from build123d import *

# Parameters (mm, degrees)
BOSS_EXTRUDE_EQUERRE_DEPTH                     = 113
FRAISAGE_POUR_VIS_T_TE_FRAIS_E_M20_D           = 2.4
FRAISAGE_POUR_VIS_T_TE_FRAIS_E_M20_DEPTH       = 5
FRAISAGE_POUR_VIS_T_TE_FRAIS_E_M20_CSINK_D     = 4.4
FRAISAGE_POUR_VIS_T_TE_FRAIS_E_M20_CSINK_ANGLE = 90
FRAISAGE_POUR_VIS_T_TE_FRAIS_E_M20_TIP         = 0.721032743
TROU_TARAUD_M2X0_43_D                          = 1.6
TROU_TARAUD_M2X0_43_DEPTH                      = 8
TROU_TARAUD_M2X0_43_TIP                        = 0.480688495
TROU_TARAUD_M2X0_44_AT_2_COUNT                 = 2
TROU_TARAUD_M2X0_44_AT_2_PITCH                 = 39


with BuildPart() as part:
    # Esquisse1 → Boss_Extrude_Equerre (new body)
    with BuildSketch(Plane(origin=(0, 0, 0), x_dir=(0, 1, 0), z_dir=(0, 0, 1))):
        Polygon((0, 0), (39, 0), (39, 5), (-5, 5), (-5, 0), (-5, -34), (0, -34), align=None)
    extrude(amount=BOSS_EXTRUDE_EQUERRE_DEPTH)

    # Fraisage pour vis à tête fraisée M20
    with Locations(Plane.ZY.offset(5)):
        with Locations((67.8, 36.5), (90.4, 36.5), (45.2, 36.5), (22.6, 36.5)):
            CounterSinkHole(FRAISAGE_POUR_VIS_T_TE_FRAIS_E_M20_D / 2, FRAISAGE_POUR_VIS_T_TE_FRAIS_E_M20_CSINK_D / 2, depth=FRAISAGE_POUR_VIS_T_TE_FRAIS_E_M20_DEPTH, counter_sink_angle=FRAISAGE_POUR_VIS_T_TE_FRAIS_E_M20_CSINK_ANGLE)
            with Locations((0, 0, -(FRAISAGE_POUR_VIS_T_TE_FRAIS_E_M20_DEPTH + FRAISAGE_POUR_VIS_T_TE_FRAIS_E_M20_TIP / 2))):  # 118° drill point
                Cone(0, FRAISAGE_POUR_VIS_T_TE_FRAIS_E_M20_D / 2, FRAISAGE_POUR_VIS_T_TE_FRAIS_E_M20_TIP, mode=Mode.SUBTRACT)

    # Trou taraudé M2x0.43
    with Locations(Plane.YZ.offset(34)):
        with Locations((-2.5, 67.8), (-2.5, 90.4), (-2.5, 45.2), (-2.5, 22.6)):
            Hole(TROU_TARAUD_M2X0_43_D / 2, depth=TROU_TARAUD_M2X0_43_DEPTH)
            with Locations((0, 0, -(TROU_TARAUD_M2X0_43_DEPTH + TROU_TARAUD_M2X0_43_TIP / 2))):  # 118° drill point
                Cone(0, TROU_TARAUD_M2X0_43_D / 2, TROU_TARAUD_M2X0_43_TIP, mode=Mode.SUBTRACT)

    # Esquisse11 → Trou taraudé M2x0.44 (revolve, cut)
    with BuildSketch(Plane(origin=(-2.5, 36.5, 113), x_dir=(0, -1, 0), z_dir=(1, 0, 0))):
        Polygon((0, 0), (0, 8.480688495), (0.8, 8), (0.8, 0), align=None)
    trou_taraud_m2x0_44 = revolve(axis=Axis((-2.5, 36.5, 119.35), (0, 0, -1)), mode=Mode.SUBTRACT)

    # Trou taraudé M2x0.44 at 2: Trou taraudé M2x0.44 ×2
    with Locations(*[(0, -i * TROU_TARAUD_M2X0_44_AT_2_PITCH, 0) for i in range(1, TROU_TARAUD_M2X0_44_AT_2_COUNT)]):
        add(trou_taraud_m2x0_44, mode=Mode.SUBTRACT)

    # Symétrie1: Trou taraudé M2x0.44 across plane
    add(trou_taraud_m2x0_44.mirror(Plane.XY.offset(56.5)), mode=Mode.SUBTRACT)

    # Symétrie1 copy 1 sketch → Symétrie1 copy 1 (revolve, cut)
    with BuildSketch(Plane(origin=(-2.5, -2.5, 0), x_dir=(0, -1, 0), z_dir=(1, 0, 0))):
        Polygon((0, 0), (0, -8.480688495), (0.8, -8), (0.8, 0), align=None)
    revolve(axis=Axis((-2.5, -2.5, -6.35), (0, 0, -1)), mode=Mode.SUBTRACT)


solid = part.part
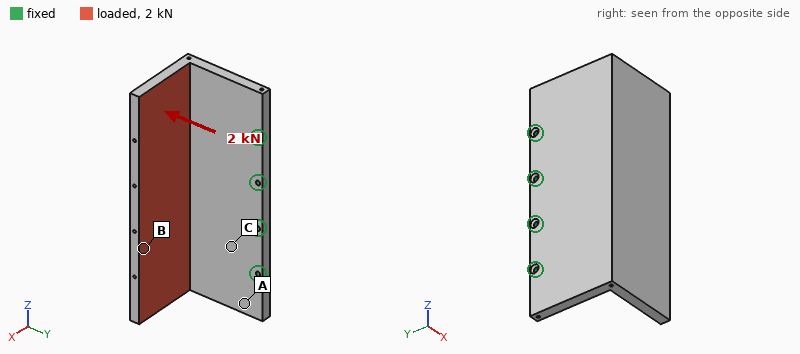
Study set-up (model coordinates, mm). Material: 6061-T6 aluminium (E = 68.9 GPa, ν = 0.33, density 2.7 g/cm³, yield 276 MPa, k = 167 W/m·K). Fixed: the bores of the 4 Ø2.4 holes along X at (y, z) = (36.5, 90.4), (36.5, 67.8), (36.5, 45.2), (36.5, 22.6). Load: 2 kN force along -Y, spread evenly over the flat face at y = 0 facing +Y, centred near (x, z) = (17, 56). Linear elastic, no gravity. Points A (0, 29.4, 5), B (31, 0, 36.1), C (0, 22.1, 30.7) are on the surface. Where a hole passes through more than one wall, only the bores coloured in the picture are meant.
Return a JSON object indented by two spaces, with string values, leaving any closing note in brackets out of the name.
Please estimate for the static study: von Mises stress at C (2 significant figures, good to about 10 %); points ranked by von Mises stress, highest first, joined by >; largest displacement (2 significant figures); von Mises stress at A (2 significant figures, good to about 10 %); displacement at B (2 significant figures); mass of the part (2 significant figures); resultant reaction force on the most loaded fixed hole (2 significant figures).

{
  "von Mises stress at C": "83 MPa",
  "points ranked by von Mises stress, highest first, joined by >": "C > A > B",
  "largest displacement": "1.1 mm",
  "von Mises stress at A": "48 MPa",
  "displacement at B": "0.98 mm",
  "mass of the part": "120 g",
  "resultant reaction force on the most loaded fixed hole": "560 N"
}
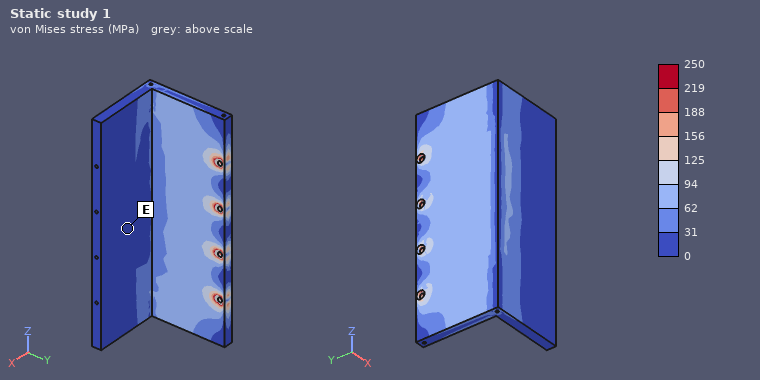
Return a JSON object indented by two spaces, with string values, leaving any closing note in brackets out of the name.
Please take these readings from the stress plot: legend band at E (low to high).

{
  "legend band at E": "0 to 31 MPa"
}
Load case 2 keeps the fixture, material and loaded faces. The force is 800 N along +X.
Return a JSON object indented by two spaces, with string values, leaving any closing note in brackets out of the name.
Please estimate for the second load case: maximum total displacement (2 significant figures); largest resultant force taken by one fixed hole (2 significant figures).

{
  "maximum total displacement": "0.48 mm",
  "largest resultant force taken by one fixed hole": "210 N"
}
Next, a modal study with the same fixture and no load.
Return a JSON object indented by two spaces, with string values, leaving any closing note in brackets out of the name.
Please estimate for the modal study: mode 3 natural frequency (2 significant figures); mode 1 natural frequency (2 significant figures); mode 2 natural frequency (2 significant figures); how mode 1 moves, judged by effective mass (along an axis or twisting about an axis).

{
  "mode 3 natural frequency": "2500 Hz",
  "mode 1 natural frequency": "770 Hz",
  "mode 2 natural frequency": "1200 Hz",
  "how mode 1 moves, judged by effective mass": "along X"
}
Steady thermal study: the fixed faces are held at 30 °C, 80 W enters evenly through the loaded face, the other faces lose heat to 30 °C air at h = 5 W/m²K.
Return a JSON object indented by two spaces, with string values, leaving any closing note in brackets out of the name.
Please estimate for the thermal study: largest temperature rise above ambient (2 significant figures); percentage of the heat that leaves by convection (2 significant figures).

{
  "largest temperature rise above ambient": "55 K",
  "percentage of the heat that leaves by convection": "3.1 %"
}
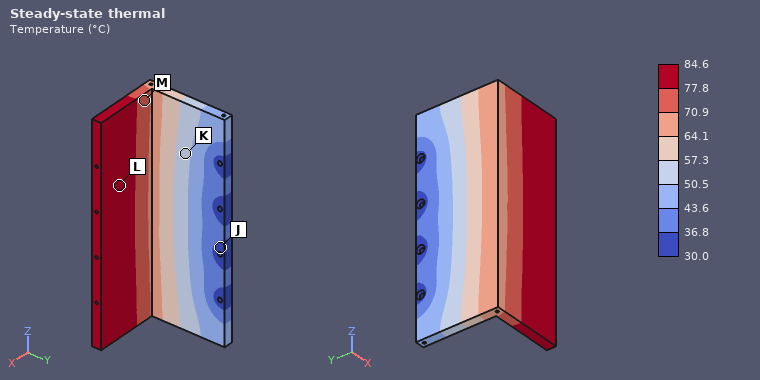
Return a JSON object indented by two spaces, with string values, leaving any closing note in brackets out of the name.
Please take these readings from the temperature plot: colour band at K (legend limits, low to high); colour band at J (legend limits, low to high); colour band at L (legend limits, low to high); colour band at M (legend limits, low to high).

{
  "colour band at K": "50.5 to 57.3 °C",
  "colour band at J": "30.0 to 36.8 °C",
  "colour band at L": "77.8 to 84.6 °C",
  "colour band at M": "70.9 to 77.8 °C"
}
